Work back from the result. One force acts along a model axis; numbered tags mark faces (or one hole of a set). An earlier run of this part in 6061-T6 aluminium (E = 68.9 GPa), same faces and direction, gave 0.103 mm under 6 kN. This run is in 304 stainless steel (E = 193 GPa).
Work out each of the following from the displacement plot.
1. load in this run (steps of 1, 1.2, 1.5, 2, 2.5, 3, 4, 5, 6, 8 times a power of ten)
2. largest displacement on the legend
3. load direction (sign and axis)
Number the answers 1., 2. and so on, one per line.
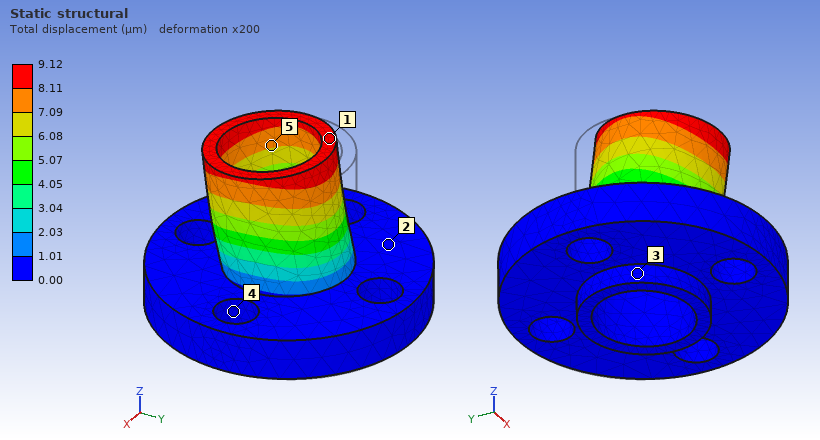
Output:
1. 1.5 kN
2. 9.12 µm
3. -Y
